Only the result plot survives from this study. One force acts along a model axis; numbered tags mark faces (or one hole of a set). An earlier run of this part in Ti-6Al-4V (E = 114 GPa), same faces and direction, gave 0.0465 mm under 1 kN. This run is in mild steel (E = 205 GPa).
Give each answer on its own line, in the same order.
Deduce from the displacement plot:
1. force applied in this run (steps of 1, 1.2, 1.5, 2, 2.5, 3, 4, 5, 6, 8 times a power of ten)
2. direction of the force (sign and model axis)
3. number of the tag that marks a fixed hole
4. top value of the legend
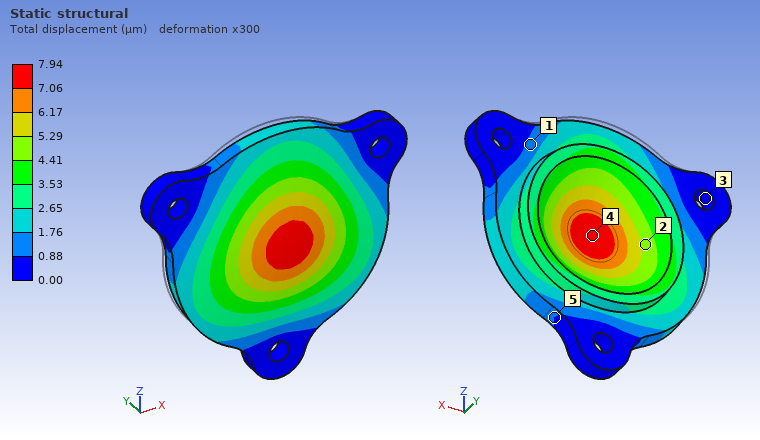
300 N
-Y
3
7.94 µm
